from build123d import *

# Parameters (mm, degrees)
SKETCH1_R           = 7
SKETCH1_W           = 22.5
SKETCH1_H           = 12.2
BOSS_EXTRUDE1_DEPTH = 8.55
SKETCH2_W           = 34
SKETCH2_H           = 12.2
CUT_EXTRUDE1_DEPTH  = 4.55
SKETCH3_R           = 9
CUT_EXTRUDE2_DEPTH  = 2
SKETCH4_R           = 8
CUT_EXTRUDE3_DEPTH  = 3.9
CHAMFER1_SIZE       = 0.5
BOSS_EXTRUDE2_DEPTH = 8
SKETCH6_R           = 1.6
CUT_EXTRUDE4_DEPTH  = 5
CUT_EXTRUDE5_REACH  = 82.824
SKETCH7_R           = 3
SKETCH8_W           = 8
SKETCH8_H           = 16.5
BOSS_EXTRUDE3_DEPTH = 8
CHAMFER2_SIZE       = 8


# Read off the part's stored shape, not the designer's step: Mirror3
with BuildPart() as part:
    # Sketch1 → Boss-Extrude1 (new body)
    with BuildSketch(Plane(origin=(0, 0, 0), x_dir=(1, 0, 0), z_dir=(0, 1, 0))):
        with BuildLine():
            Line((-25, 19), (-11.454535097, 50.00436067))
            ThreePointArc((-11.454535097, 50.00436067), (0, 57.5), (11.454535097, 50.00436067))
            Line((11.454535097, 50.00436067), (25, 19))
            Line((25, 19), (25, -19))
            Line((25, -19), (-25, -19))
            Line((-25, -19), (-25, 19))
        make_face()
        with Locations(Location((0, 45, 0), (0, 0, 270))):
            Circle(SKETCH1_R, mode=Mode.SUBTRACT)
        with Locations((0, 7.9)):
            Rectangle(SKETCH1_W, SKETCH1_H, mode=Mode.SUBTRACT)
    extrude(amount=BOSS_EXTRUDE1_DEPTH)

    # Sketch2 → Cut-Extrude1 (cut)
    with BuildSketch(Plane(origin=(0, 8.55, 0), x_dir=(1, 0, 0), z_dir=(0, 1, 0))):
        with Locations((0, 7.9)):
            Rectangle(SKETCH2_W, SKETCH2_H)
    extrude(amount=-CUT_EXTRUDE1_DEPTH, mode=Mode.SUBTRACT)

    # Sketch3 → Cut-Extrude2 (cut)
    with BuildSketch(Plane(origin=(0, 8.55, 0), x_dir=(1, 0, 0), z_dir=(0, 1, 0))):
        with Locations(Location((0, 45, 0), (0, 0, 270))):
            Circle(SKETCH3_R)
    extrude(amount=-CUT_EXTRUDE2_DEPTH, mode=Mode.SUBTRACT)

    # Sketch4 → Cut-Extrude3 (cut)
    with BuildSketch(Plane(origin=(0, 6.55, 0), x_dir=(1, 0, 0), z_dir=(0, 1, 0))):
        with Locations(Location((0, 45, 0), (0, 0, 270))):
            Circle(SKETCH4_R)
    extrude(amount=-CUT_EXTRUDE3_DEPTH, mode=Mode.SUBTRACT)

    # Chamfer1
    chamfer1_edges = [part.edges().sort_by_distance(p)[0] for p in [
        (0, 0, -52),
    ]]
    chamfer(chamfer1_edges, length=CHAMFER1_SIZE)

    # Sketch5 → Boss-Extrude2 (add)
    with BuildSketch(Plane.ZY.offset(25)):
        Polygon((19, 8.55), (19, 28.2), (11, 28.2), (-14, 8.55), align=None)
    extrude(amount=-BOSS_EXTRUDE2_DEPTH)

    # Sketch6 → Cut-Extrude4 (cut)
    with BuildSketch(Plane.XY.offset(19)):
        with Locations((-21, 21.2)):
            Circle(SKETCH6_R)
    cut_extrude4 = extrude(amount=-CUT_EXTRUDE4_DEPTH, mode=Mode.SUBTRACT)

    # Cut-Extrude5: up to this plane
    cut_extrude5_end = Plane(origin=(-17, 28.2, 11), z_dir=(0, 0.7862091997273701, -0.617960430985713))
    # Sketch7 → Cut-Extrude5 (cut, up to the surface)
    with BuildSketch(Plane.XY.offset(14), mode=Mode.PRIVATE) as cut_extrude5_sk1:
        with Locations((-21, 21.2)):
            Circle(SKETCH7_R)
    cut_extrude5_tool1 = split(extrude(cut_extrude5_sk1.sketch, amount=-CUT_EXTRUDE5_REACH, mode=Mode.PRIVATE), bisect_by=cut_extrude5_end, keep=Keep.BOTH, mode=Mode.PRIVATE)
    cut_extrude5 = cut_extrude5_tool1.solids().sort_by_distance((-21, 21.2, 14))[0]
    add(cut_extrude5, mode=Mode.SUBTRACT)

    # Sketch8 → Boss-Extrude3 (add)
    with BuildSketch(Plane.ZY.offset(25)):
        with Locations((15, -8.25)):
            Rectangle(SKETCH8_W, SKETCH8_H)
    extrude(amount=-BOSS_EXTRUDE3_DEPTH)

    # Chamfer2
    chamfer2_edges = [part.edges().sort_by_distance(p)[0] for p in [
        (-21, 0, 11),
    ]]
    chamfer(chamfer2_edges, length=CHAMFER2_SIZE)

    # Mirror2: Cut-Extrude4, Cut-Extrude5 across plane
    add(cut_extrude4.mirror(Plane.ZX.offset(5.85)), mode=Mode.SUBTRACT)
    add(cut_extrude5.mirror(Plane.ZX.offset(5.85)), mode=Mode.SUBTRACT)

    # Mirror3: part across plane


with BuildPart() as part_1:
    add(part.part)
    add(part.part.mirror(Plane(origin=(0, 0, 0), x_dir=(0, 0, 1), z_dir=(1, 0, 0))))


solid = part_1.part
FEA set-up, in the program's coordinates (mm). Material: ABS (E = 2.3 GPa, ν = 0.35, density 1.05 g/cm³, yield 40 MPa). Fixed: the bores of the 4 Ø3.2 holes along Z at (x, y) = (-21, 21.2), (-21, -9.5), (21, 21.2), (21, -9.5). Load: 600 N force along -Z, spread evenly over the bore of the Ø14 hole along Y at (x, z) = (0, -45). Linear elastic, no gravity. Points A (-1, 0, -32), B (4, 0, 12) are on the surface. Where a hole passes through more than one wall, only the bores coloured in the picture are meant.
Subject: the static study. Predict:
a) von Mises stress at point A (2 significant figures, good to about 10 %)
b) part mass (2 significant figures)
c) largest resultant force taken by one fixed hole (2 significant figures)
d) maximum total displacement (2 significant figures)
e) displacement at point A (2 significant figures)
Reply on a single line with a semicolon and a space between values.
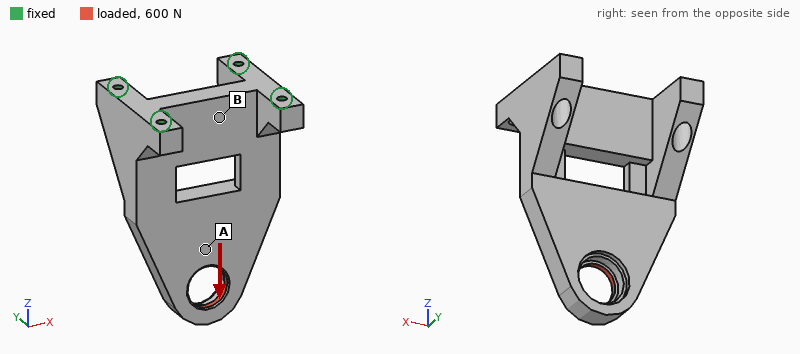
4.7 MPa; 32 g; 220 N; 0.88 mm; 0.35 mm
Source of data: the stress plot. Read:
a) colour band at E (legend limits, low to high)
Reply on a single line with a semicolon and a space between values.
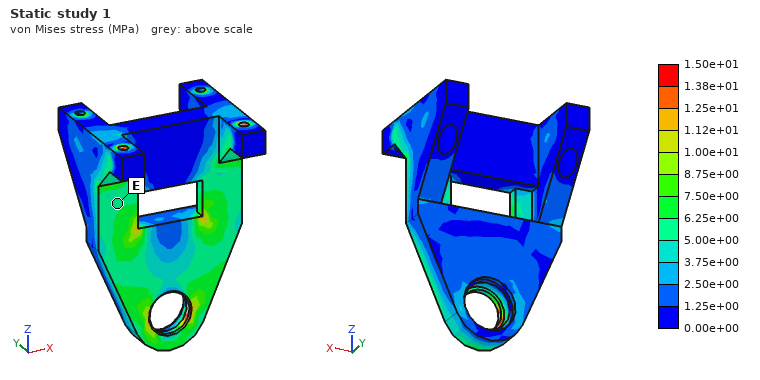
5.00e+00 to 6.25e+00 MPa
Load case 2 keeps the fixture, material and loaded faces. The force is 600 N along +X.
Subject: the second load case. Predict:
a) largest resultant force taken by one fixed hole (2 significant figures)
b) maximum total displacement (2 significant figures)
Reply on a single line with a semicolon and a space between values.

510 N; 0.94 mm
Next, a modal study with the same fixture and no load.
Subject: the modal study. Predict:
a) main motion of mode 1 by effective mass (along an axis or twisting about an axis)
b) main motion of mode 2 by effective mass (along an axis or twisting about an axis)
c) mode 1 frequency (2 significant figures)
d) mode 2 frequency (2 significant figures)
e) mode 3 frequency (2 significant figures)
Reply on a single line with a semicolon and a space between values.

along Y; along X; 790 Hz; 1400 Hz; 2500 Hz
